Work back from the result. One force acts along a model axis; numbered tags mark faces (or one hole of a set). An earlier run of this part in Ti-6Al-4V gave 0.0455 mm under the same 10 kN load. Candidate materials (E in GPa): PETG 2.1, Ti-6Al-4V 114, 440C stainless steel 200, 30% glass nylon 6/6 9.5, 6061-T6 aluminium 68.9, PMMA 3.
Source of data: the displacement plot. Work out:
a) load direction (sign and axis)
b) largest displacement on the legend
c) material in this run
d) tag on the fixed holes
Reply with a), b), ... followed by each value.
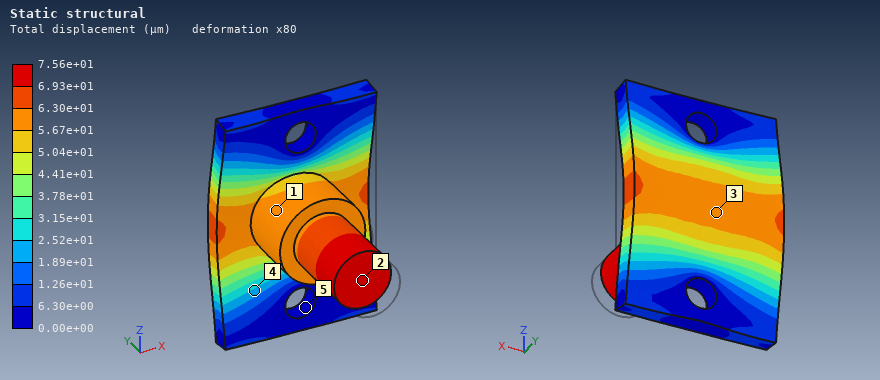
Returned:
a) +Y
b) 7.56e+01 µm
c) 6061-T6 aluminium
d) 5
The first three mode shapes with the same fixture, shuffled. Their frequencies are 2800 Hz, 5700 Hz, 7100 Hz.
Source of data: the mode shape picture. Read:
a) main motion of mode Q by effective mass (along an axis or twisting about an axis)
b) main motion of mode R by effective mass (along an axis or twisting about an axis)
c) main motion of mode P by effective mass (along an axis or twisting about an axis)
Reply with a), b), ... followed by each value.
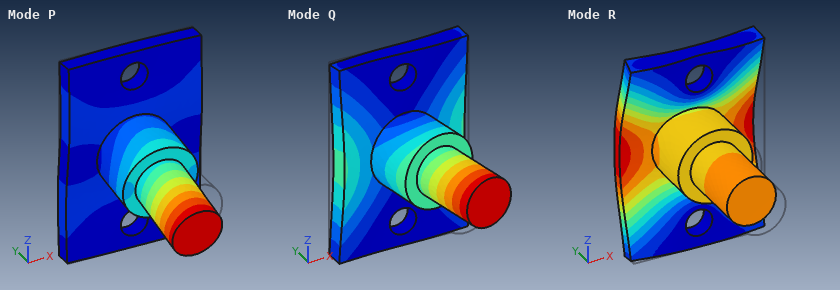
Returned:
a) along X
b) along Y
c) along Z
